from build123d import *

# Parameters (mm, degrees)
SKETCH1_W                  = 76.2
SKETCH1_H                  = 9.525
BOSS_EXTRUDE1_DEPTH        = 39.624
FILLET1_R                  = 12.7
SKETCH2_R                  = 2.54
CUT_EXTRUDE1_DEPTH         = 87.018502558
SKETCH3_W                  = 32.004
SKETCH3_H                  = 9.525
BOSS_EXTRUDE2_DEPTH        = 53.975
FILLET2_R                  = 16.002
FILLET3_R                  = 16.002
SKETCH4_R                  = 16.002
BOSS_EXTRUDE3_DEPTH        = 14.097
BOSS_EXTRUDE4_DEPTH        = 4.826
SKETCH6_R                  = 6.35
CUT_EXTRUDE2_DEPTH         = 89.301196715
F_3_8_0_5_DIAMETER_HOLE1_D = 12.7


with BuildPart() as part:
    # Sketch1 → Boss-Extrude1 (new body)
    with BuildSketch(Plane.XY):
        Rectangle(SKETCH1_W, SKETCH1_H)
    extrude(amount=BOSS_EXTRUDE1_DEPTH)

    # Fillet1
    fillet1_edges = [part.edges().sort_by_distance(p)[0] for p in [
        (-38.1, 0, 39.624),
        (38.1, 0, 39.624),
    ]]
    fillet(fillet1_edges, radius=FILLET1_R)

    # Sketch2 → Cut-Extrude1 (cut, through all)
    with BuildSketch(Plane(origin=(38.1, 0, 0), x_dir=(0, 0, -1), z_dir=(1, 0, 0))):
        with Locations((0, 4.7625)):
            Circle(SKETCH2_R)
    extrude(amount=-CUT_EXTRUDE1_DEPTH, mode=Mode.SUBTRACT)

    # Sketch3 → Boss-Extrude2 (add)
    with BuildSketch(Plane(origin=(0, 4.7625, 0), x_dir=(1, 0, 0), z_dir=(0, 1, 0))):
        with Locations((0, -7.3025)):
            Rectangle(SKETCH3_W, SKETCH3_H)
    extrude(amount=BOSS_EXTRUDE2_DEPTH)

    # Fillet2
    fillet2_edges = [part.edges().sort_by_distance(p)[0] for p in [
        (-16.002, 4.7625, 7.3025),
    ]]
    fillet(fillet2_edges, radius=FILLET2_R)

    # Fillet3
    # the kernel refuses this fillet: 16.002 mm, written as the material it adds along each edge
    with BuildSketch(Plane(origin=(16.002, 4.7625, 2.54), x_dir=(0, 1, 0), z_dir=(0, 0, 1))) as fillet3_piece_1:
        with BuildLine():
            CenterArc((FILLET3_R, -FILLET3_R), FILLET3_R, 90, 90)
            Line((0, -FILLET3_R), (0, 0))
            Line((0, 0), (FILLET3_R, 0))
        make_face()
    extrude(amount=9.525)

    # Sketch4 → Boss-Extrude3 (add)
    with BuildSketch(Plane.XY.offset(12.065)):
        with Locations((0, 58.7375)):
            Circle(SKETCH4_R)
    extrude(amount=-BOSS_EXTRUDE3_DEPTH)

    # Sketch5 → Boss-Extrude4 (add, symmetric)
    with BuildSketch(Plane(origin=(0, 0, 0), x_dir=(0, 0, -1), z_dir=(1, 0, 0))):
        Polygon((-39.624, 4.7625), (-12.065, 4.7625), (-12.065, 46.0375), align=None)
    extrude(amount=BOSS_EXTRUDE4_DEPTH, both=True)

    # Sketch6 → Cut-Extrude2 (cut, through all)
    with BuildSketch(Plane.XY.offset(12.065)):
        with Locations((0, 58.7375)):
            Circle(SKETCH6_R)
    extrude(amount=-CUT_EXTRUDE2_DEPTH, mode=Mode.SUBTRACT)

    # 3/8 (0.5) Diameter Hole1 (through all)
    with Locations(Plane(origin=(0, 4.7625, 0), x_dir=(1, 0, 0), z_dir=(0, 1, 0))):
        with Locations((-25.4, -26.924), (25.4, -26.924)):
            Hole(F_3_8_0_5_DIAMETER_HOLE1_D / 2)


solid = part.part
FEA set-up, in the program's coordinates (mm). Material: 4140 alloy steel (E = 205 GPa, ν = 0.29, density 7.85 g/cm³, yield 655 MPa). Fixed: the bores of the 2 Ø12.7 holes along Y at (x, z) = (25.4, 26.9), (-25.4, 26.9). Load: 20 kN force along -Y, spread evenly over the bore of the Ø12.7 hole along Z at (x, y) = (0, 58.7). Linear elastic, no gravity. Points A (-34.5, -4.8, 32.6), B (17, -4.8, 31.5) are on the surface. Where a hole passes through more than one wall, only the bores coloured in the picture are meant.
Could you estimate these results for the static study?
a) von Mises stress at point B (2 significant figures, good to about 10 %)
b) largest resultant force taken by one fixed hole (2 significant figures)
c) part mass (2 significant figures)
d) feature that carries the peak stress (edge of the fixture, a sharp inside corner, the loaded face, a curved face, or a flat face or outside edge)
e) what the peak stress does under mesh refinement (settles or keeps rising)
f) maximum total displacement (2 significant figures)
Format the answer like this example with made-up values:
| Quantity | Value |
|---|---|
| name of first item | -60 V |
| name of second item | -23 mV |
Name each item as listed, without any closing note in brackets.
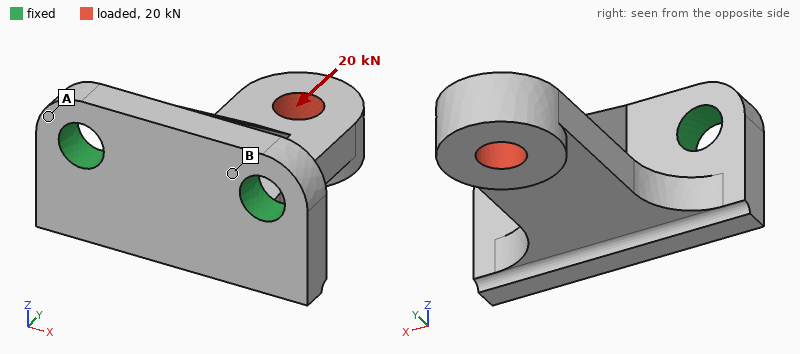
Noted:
| Quantity | Value |
|---|---|
| von Mises stress at point B | 140 MPa |
| largest resultant force taken by one fixed hole | 10 kN |
| part mass | 420 g |
| feature that carries the peak stress | edge of the fixture |
| what the peak stress does under mesh refinement | keeps rising |
| maximum total displacement | 0.28 mm |
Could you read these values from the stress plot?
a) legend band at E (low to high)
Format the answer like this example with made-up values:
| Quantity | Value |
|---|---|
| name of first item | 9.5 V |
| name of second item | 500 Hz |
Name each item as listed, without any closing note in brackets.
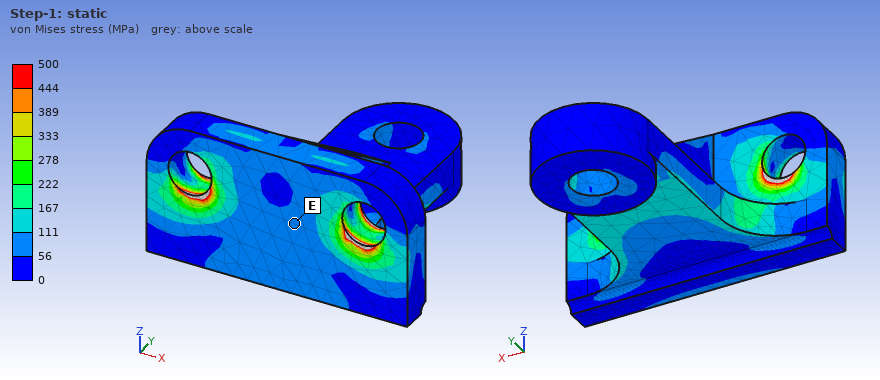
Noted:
| Quantity | Value |
|---|---|
| legend band at E | 56 to 111 MPa |
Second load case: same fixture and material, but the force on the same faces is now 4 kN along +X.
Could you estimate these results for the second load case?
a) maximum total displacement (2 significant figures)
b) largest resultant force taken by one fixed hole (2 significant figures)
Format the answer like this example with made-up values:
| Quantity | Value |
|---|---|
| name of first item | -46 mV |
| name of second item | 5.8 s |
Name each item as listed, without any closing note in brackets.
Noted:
| Quantity | Value |
|---|---|
| maximum total displacement | 100 µm |
| largest resultant force taken by one fixed hole | 5.7 kN |
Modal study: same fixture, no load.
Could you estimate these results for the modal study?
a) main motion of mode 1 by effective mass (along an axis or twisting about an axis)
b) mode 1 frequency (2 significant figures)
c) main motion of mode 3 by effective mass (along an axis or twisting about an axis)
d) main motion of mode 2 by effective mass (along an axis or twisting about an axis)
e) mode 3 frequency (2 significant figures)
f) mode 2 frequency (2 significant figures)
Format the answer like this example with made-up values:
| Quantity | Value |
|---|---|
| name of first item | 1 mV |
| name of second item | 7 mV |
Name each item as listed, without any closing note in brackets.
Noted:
| Quantity | Value |
|---|---|
| main motion of mode 1 by effective mass | along Z |
| mode 1 frequency | 2300 Hz |
| main motion of mode 3 by effective mass | along Y |
| main motion of mode 2 by effective mass | along X |
| mode 3 frequency | 7400 Hz |
| mode 2 frequency | 3700 Hz |
